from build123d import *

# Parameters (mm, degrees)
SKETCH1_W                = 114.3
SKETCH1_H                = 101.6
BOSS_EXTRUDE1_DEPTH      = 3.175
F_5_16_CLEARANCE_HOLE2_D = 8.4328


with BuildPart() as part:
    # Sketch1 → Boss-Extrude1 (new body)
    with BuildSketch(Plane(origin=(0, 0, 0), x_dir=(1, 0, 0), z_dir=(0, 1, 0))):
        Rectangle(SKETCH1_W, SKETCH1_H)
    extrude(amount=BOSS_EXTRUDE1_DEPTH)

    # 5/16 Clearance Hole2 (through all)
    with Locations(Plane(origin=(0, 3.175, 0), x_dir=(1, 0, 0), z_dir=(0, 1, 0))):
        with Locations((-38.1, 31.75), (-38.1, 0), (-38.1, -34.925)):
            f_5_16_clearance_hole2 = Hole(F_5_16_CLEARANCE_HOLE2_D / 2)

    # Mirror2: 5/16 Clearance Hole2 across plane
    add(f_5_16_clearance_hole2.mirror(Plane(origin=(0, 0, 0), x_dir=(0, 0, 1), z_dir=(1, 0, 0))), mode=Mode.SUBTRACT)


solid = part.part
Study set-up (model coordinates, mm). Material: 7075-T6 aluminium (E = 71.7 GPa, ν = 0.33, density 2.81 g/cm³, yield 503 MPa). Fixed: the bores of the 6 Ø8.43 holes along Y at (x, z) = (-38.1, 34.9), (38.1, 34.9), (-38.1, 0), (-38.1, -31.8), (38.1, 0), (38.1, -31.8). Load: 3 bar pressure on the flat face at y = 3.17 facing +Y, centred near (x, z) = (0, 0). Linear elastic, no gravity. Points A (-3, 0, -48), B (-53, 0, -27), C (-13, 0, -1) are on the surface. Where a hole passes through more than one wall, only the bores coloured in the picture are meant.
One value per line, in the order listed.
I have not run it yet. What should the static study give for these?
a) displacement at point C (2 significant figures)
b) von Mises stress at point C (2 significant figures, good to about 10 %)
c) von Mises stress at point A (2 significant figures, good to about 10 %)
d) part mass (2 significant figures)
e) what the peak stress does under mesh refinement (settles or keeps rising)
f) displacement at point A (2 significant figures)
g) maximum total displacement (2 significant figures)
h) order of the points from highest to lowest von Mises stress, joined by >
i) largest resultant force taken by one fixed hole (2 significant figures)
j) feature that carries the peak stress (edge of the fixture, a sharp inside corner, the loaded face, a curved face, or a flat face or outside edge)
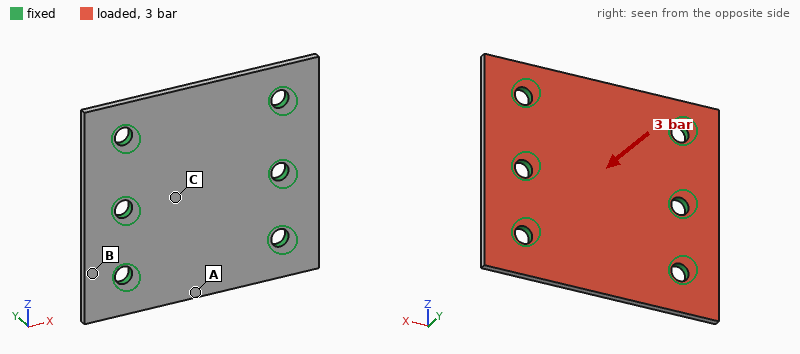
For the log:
0.081 mm
23 MPa
38 MPa
100 g
keeps rising
0.14 mm
0.14 mm
A > C > B
590 N
edge of the fixture
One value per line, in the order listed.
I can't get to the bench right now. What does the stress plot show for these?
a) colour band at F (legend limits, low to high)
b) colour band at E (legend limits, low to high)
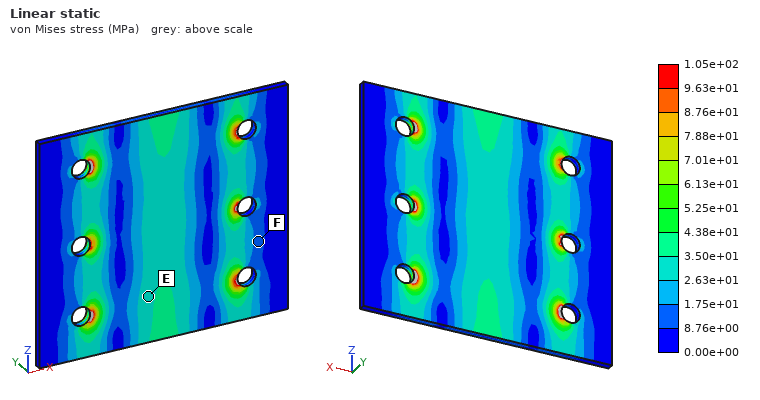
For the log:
8.76e+00 to 1.75e+01 MPa
2.63e+01 to 3.50e+01 MPa
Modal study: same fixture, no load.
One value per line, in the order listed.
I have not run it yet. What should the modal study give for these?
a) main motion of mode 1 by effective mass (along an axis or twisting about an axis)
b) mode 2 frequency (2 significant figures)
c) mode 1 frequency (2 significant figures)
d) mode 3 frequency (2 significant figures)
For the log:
along Y
3300 Hz
3100 Hz
4300 Hz
